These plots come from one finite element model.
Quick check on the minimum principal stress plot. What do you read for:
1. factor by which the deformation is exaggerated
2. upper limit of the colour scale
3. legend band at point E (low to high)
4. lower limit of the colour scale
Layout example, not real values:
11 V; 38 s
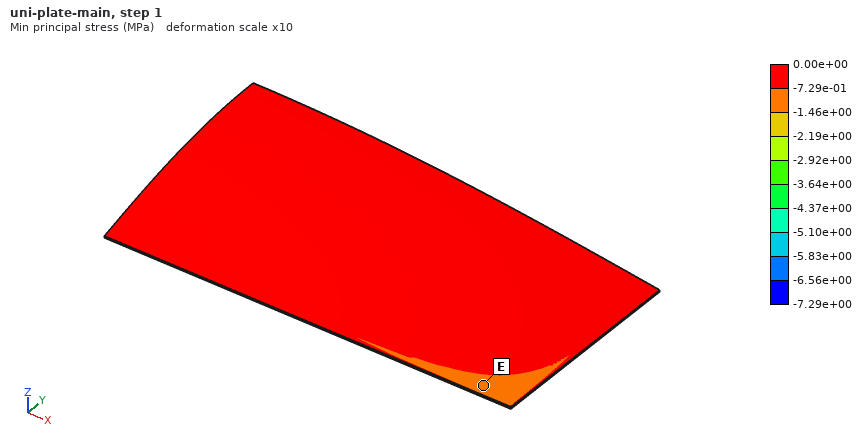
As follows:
10; 0.00e+00 MPa; -1.46e+00 to -7.29e-01 MPa; -7.29e+00 MPa
